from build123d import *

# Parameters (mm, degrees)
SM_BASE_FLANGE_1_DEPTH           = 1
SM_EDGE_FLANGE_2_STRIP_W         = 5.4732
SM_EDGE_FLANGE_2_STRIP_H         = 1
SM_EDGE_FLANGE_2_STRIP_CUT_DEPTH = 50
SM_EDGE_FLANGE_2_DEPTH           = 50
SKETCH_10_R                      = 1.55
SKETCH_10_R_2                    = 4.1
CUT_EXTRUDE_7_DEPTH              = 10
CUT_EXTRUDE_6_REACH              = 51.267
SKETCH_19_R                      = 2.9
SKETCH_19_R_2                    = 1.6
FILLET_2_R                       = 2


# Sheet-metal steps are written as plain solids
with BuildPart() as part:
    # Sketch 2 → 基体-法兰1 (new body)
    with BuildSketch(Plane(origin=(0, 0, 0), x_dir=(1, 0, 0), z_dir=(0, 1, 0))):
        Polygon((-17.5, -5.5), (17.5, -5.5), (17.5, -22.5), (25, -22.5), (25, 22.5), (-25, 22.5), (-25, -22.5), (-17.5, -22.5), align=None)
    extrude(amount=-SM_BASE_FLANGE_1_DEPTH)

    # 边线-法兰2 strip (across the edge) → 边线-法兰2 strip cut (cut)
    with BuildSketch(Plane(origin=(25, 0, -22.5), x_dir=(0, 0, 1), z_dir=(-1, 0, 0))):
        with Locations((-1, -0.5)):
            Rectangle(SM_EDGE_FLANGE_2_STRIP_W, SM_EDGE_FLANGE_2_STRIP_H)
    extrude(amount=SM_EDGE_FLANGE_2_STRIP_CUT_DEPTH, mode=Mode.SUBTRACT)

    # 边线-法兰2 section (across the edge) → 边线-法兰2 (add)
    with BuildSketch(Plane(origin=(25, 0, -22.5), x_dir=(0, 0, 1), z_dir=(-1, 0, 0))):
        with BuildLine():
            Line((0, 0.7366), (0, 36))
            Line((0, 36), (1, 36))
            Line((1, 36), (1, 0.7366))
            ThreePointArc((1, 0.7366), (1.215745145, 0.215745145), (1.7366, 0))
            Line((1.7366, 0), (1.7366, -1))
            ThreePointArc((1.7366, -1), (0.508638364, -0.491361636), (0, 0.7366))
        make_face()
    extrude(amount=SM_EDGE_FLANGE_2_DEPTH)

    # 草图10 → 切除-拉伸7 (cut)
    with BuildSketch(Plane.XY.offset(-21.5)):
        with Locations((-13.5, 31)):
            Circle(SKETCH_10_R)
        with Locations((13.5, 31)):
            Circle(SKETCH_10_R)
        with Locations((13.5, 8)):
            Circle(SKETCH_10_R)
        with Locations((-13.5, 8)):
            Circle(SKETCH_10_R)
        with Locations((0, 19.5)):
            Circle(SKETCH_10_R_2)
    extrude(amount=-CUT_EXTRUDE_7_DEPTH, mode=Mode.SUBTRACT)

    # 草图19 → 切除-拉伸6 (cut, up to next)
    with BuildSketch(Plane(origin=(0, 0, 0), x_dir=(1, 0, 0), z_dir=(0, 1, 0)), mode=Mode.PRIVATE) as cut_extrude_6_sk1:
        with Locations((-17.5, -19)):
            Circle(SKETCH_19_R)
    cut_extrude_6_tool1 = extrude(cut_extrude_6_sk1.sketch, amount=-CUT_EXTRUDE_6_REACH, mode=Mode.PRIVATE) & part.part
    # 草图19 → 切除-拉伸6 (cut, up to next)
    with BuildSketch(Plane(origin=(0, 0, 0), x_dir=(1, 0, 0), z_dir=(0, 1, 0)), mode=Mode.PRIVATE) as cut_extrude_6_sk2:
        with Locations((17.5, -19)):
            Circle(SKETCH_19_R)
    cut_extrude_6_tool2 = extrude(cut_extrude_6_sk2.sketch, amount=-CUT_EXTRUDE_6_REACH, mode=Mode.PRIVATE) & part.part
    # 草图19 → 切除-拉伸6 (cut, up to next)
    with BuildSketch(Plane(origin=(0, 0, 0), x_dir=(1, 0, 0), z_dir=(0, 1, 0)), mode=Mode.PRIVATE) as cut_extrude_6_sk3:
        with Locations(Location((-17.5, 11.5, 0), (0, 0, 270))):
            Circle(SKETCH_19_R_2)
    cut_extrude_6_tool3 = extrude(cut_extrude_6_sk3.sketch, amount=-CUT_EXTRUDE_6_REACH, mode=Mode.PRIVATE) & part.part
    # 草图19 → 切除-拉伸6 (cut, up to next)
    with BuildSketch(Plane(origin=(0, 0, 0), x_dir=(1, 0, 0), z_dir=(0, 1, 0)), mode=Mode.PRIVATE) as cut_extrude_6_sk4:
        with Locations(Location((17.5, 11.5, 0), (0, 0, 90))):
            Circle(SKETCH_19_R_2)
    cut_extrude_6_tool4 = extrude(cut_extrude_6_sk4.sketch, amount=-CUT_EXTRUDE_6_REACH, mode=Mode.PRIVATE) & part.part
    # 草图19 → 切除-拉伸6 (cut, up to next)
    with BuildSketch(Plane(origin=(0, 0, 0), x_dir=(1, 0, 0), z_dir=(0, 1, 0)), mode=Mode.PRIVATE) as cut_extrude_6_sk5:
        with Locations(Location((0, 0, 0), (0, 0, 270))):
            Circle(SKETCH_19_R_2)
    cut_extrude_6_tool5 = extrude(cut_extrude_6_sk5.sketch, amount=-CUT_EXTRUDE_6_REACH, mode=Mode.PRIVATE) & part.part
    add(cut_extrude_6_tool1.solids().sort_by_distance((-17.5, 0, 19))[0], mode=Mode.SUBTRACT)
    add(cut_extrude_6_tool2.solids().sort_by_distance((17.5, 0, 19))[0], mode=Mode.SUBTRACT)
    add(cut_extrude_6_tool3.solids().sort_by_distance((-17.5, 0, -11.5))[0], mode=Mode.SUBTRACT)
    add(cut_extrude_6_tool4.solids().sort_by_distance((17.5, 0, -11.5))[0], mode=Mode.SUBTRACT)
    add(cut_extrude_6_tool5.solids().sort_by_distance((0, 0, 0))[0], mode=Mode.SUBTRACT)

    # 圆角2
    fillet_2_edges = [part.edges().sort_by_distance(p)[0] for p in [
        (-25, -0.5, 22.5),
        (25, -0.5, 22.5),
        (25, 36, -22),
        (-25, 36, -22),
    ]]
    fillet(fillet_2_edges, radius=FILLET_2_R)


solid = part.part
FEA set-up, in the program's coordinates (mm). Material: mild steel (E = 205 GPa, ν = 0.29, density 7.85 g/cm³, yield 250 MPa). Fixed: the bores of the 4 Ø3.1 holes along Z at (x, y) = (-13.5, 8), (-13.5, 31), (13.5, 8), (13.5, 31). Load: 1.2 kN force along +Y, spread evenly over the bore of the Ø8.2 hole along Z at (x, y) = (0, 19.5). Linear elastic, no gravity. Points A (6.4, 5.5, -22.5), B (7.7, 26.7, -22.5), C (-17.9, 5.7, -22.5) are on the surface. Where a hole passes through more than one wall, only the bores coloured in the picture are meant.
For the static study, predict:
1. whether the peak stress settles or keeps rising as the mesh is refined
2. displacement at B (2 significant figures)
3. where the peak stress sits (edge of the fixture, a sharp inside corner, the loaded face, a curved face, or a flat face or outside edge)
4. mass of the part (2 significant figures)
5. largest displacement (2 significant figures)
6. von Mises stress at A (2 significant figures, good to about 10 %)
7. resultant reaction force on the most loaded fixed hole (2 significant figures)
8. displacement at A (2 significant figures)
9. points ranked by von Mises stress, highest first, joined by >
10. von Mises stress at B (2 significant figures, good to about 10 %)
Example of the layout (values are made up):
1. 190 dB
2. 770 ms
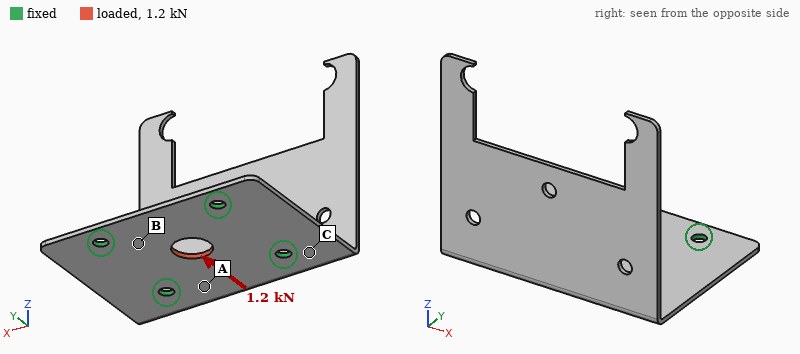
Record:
1. keeps rising
2. 1.7 µm
3. edge of the fixture
4. 26 g
5. 3.8 µm
6. 21 MPa
7. 340 N
8. 1.6 µm
9. B > A > C
10. 38 MPa
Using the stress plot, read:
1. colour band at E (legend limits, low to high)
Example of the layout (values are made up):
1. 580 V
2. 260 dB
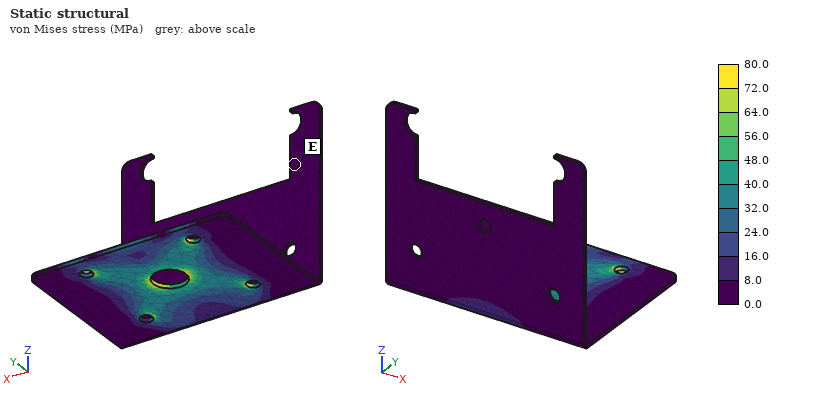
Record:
1. 0.0 to 8.0 MPa
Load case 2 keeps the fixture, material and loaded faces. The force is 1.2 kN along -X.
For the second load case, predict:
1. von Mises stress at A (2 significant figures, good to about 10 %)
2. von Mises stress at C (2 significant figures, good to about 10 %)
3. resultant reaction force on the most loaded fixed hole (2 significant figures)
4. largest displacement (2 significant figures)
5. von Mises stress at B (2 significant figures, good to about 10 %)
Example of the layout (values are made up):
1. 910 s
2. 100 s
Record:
1. 8.3 MPa
2. 6.5 MPa
3. 320 N
4. 2.8 µm
5. 33 MPa
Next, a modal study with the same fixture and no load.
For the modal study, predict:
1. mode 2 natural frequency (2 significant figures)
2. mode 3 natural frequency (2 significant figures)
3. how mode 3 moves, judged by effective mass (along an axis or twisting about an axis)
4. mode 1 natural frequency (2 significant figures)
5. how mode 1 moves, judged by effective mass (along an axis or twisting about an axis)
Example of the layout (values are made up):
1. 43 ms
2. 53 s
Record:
1. 810 Hz
2. 1900 Hz
3. along X
4. 510 Hz
5. along Y
